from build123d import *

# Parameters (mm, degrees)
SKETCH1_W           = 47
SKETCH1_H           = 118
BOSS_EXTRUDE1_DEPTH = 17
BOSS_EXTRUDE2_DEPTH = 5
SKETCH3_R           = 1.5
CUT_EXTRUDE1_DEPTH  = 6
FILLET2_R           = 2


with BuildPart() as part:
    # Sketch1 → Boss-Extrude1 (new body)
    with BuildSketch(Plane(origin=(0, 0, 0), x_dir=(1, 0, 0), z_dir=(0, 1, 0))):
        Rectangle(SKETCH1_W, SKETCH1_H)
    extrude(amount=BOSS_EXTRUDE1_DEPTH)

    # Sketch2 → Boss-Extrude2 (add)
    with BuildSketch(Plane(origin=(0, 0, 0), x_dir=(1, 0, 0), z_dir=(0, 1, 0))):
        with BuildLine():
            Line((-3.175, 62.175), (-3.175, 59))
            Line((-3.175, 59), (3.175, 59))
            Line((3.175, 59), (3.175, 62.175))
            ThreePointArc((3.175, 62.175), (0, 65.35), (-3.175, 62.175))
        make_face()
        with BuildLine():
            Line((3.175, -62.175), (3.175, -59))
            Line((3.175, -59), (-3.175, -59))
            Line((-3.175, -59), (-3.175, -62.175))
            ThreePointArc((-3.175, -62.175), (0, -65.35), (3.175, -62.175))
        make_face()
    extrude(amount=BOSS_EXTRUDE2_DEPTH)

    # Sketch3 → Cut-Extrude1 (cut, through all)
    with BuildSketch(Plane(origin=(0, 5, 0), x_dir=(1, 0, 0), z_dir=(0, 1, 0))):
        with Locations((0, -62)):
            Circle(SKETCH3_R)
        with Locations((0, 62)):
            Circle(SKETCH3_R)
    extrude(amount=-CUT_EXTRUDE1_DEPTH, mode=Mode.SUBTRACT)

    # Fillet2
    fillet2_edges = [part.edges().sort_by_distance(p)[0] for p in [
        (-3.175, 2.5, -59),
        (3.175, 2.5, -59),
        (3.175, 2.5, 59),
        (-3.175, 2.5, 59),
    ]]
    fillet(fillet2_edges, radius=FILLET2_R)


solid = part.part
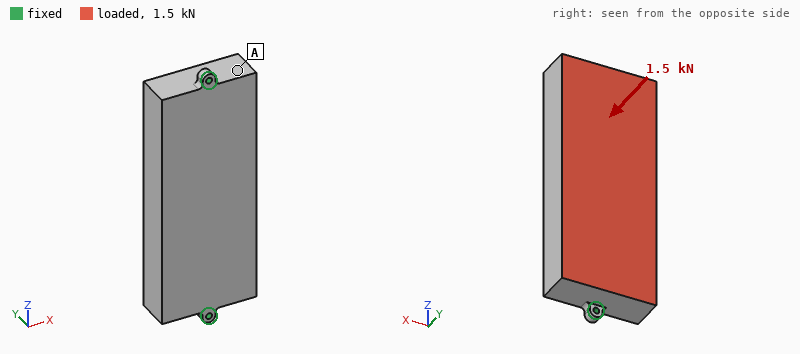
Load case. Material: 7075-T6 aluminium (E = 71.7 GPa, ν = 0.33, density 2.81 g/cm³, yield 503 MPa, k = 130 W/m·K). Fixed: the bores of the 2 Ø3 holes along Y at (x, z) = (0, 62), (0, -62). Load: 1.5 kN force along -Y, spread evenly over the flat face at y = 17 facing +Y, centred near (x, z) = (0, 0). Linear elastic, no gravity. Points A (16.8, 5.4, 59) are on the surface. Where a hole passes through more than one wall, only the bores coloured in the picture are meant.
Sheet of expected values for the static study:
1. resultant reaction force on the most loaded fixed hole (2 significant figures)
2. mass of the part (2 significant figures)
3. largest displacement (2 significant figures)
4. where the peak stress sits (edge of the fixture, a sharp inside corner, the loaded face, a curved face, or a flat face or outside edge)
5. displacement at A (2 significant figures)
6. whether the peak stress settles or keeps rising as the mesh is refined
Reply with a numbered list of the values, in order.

1. 1.1 kN
2. 270 g
3. 24 µm
4. edge of the fixture
5. 5.4 µm
6. keeps rising
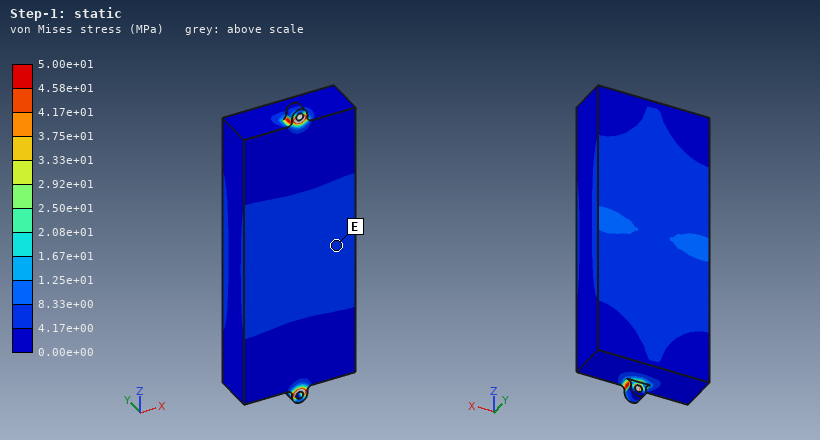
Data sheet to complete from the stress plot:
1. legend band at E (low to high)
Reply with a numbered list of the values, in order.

1. 4.17e+00 to 8.33e+00 MPa
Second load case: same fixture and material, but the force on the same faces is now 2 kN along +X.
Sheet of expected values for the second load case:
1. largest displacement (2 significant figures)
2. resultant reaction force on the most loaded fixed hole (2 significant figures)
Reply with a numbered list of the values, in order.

1. 0.30 mm
2. 1.0 kN
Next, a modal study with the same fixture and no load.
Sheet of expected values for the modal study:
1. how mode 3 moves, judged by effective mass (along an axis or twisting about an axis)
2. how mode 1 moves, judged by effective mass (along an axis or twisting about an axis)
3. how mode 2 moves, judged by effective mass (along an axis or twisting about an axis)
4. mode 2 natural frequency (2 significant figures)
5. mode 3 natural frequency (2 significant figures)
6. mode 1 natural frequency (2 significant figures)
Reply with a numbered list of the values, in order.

1. along X
2. along X
3. along Y
4. 2800 Hz
5. 4900 Hz
6. 1000 Hz
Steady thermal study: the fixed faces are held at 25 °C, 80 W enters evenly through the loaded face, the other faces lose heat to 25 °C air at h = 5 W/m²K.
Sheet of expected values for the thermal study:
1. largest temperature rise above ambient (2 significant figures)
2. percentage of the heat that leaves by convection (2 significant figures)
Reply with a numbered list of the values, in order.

1. 53 K
2. 3.3 %
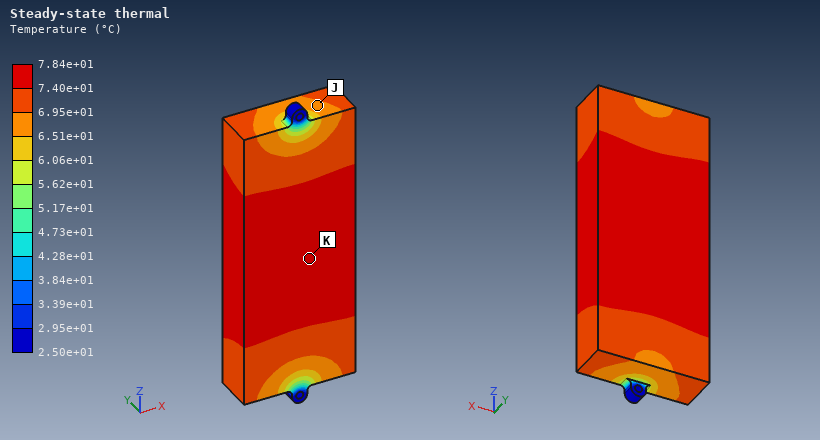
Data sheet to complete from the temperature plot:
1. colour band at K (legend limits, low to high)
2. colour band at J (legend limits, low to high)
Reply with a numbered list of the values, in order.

1. 7.40e+01 to 7.84e+01 °C
2. 6.51e+01 to 6.95e+01 °C
